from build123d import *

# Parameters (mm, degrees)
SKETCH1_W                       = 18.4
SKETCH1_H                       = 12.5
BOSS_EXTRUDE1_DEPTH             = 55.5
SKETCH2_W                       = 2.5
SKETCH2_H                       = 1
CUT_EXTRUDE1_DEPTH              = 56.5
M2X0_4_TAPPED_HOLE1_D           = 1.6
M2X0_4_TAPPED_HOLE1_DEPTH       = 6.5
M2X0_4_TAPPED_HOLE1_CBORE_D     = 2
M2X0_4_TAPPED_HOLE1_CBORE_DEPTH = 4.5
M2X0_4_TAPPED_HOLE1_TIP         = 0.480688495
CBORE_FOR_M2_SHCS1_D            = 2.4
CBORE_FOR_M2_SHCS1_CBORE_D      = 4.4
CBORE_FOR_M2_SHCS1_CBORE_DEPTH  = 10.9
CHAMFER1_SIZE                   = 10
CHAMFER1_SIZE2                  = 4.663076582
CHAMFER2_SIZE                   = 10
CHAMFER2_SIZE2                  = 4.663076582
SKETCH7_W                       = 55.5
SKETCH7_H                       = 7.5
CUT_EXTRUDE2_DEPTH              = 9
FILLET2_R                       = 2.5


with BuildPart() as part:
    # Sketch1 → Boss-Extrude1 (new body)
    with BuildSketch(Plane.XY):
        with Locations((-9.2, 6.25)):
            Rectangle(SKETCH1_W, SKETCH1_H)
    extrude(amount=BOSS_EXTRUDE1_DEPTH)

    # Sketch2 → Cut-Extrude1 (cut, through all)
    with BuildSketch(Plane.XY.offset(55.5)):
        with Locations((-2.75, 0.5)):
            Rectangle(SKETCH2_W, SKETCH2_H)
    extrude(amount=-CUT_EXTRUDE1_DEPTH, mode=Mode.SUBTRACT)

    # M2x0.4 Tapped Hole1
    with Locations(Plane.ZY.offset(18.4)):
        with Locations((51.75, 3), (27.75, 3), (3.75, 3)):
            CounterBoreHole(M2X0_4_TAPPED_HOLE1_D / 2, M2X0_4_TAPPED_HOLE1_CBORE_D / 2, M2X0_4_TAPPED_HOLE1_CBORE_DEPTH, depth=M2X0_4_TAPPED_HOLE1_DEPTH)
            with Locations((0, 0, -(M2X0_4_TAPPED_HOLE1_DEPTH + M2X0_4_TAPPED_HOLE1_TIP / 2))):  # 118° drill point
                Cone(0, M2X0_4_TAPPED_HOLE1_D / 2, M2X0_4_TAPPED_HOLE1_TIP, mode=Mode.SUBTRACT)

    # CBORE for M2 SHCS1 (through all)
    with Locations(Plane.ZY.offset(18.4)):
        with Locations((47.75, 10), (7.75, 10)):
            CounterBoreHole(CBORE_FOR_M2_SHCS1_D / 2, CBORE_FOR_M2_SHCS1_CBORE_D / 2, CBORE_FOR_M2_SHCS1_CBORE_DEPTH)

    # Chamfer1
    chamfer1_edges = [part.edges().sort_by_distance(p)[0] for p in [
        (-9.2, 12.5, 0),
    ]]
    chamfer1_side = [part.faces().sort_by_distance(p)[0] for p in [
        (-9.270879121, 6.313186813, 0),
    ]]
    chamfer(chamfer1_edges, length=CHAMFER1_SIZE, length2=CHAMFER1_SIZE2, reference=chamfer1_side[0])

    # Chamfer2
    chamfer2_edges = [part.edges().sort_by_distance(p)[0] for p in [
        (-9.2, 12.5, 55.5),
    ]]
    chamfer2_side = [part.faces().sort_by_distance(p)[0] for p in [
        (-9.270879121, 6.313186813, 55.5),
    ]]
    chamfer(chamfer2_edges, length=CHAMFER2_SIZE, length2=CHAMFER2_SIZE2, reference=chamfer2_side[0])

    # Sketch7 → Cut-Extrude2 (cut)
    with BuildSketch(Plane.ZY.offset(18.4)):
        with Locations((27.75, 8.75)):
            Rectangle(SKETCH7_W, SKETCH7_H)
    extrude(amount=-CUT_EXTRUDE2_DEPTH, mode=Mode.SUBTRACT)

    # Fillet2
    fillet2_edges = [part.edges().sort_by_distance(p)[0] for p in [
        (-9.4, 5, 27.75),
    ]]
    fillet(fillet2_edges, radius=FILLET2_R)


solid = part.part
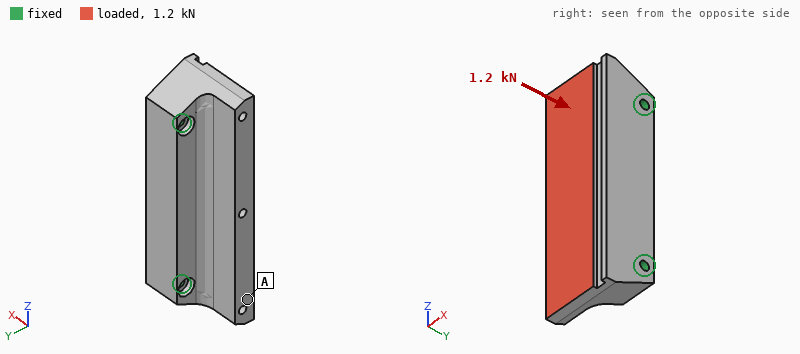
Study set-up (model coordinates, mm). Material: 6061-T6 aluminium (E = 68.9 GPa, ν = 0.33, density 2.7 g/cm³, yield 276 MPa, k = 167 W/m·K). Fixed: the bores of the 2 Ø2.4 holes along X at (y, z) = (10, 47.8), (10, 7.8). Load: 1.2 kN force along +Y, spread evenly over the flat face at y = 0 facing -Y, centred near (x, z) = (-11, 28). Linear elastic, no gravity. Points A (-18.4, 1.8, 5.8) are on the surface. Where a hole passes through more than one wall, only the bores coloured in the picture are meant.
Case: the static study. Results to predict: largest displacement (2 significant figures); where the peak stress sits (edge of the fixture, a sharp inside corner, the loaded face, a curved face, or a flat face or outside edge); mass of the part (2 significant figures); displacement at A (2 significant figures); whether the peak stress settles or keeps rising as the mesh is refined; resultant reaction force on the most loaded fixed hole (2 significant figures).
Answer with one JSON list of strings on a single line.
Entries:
["25 µm", "edge of the fixture", "22 g", "17 µm", "keeps rising", "650 N"]
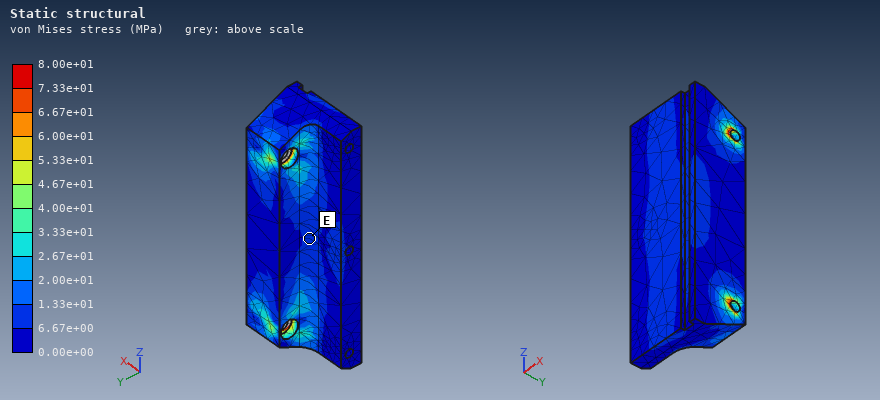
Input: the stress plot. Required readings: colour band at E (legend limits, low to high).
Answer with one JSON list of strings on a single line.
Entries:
["6.67e+00 to 1.33e+01 MPa"]
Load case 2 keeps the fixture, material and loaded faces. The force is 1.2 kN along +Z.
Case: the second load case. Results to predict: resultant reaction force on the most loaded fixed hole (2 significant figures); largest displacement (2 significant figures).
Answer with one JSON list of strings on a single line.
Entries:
["690 N", "5.1 µm"]
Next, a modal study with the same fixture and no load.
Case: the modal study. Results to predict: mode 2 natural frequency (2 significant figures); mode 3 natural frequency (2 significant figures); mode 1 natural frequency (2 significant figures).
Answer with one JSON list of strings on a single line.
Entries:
["20 kHz", "20 kHz", "11 kHz"]
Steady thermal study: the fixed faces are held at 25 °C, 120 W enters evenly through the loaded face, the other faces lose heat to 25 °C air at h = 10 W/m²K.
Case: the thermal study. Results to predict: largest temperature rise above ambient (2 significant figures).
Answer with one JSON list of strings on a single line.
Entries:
["42 K"]
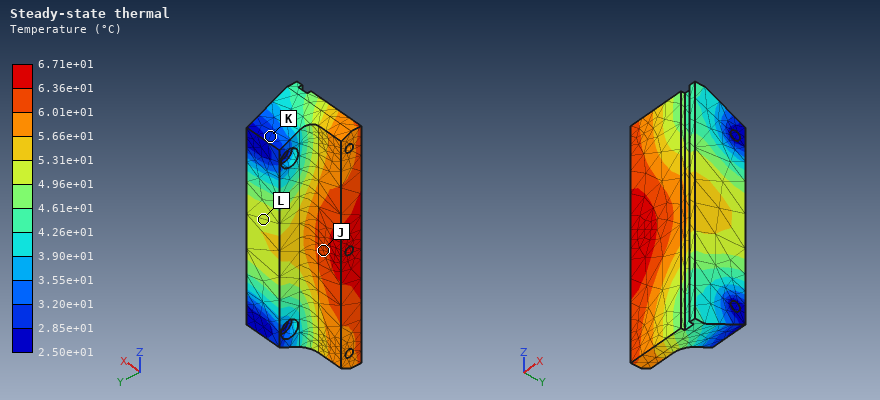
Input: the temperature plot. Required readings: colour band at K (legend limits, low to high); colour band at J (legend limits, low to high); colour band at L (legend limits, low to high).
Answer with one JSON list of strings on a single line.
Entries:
["2.85e+01 to 3.20e+01 °C", "6.01e+01 to 6.36e+01 °C", "4.96e+01 to 5.31e+01 °C"]
